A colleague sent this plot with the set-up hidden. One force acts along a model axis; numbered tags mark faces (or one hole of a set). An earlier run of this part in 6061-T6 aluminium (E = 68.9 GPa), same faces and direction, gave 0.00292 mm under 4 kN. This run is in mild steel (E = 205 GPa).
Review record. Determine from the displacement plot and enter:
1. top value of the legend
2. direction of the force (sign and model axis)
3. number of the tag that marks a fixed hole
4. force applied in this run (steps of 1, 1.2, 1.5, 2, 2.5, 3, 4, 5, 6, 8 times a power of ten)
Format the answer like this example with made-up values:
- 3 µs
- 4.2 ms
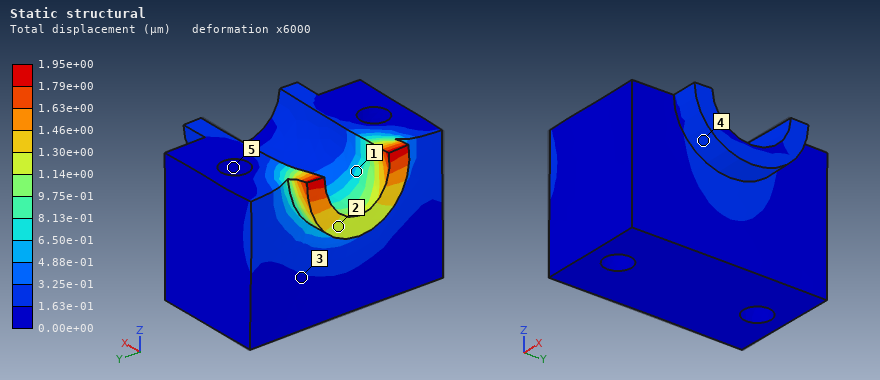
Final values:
- 1.95e+00 µm
- +X
- 5
- 8 kN
